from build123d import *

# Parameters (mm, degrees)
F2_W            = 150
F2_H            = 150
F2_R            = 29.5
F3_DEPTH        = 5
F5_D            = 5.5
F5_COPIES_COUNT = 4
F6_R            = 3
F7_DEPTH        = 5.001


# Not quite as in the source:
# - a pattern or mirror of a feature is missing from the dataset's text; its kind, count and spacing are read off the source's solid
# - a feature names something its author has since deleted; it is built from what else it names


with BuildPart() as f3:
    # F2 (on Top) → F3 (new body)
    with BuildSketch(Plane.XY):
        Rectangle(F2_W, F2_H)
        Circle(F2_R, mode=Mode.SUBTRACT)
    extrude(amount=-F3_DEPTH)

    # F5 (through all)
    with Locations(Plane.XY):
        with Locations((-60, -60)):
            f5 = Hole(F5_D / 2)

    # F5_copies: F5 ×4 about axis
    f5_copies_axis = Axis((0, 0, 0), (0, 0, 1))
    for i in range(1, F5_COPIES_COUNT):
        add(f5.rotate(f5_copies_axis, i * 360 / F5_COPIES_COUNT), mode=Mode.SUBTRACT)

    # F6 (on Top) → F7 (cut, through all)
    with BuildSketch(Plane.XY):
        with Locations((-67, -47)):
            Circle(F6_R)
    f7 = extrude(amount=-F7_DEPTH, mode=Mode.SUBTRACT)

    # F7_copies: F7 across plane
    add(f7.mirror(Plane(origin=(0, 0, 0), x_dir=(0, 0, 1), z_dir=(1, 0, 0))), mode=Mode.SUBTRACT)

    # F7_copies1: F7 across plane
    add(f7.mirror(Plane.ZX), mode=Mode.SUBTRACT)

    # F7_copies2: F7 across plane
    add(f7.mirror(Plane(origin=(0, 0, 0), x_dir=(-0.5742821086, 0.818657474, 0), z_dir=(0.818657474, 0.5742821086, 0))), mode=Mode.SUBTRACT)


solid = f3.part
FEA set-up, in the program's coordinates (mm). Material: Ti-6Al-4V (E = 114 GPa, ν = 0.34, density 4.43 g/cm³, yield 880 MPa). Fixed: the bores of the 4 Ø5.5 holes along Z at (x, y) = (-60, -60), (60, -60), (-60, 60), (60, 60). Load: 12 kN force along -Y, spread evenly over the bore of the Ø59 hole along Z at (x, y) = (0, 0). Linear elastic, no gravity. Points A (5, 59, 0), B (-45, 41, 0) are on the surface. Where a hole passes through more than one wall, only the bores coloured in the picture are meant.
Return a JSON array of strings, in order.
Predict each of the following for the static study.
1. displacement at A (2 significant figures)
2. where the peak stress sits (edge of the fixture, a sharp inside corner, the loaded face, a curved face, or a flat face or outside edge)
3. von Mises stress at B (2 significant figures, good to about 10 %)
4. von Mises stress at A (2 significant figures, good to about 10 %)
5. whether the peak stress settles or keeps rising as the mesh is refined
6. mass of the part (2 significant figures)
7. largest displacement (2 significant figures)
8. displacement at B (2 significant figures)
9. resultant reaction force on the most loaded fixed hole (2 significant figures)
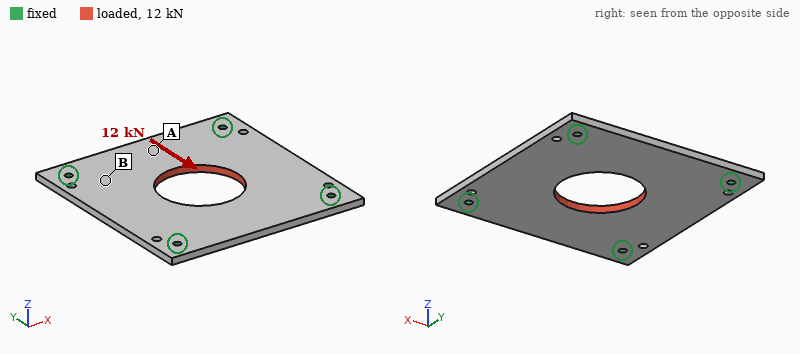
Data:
["14 µm", "edge of the fixture", "18 MPa", "6.6 MPa", "keeps rising", "430 g", "16 µm", "6.7 µm", "3.3 kN"]
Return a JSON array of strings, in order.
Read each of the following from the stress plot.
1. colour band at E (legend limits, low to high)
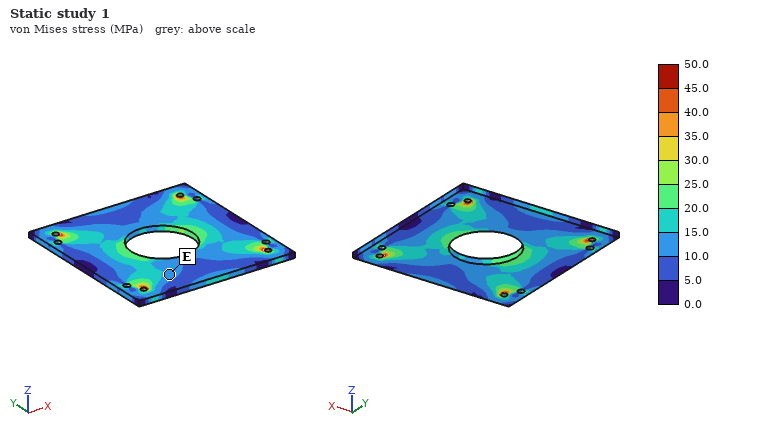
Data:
["10.0 to 15.0 MPa"]
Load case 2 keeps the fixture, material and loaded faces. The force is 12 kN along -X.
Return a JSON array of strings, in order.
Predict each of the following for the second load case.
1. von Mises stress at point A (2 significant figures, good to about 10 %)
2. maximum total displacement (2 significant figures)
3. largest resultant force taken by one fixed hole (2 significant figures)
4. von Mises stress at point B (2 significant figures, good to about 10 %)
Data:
["10 MPa", "16 µm", "3.3 kN", "18 MPa"]
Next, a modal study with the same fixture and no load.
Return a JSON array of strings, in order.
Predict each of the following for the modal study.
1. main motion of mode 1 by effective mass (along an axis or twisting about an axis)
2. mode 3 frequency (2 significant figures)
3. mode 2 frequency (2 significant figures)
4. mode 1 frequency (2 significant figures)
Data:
["along Z", "1900 Hz", "1900 Hz", "1300 Hz"]
